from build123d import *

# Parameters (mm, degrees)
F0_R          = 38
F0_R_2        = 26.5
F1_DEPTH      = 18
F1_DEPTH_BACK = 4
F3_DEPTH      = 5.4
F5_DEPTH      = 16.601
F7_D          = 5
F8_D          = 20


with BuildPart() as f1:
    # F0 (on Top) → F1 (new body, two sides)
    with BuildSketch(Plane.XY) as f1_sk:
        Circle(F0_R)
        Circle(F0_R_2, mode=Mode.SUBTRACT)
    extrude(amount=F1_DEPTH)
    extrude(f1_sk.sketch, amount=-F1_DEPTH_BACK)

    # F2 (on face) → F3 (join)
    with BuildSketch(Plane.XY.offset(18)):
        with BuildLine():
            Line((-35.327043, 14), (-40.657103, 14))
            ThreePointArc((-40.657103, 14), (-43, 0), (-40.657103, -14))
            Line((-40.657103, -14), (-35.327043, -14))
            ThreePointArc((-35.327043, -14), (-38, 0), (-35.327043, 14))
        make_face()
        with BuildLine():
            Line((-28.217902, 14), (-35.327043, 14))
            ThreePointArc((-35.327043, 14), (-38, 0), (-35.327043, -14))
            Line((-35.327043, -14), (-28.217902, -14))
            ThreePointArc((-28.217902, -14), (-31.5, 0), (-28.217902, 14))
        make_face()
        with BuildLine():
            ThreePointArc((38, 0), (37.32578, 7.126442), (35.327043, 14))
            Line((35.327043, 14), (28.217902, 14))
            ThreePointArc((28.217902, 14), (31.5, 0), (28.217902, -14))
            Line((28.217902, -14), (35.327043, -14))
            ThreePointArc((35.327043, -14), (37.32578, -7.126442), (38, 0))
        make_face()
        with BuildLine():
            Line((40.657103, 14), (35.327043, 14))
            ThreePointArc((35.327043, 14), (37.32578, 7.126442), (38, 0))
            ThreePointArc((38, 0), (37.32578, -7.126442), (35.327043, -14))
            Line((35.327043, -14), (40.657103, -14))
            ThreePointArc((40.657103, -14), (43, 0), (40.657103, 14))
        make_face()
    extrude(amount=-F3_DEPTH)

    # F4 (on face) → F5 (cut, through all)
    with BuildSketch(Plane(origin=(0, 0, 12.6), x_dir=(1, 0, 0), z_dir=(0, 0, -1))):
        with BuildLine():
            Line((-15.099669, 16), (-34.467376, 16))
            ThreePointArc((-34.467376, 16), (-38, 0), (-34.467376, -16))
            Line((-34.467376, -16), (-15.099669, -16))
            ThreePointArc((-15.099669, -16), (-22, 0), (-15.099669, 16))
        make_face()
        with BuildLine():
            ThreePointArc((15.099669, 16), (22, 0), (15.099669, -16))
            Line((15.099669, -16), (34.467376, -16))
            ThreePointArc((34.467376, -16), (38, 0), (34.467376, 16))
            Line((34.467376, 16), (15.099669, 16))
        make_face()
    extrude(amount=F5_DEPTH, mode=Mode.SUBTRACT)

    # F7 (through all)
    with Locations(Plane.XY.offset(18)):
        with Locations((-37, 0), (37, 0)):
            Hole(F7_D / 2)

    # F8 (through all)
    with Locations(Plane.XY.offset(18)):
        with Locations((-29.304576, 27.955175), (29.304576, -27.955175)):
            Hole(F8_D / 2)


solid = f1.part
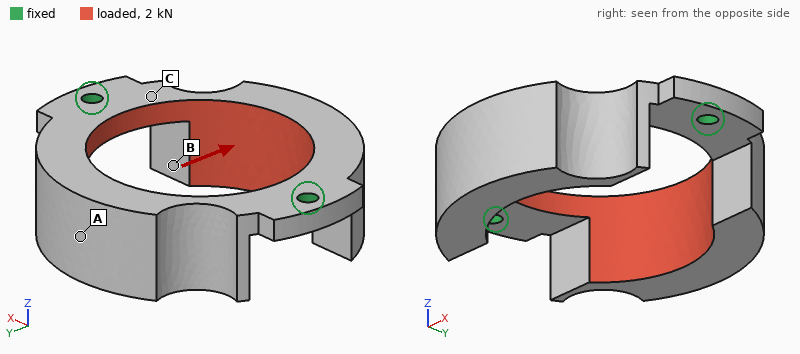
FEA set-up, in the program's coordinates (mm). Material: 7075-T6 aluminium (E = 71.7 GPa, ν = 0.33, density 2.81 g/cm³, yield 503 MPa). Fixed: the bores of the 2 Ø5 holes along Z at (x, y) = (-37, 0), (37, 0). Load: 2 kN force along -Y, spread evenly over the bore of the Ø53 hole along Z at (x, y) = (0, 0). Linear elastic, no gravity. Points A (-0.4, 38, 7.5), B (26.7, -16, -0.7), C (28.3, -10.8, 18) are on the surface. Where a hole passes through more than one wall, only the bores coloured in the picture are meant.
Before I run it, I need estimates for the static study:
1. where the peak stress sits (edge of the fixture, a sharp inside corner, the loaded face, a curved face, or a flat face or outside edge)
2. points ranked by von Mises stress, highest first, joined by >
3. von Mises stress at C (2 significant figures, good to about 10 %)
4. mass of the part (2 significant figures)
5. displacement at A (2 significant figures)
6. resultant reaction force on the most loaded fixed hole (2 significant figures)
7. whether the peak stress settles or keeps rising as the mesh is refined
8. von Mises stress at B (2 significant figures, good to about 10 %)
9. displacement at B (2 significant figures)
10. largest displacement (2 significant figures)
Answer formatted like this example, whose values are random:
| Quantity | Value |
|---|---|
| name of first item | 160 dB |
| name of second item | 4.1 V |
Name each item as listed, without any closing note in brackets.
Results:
| Quantity | Value |
|---|---|
| where the peak stress sits | edge of the fixture |
| points ranked by von Mises stress, highest first, joined by > | C > B > A |
| von Mises stress at C | 38 MPa |
| mass of the part | 99 g |
| displacement at A | 0.20 mm |
| resultant reaction force on the most loaded fixed hole | 1.0 kN |
| whether the peak stress settles or keeps rising as the mesh is refined | keeps rising |
| von Mises stress at B | 15 MPa |
| displacement at B | 0.11 mm |
| largest displacement | 0.23 mm |
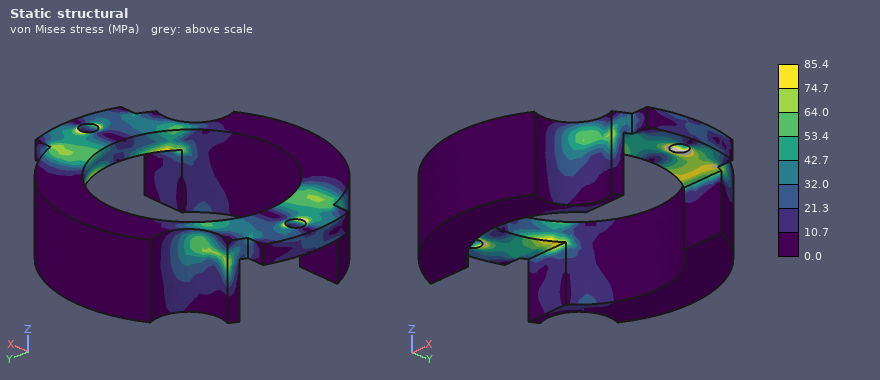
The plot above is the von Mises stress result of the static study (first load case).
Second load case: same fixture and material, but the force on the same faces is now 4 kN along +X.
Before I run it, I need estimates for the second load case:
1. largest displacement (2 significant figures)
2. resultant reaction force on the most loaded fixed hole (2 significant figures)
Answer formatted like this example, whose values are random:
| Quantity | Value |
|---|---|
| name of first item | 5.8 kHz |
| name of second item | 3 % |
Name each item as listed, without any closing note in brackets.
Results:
| Quantity | Value |
|---|---|
| largest displacement | 44 µm |
| resultant reaction force on the most loaded fixed hole | 2.0 kN |
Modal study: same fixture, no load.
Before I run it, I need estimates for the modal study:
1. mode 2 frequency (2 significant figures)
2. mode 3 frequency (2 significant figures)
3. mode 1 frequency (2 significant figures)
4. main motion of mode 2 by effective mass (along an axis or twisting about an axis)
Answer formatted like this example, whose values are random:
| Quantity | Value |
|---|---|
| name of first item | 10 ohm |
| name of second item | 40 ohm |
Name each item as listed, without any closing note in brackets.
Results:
| Quantity | Value |
|---|---|
| mode 2 frequency | 1200 Hz |
| mode 3 frequency | 5000 Hz |
| mode 1 frequency | 1200 Hz |
| main motion of mode 2 by effective mass | along Z |
